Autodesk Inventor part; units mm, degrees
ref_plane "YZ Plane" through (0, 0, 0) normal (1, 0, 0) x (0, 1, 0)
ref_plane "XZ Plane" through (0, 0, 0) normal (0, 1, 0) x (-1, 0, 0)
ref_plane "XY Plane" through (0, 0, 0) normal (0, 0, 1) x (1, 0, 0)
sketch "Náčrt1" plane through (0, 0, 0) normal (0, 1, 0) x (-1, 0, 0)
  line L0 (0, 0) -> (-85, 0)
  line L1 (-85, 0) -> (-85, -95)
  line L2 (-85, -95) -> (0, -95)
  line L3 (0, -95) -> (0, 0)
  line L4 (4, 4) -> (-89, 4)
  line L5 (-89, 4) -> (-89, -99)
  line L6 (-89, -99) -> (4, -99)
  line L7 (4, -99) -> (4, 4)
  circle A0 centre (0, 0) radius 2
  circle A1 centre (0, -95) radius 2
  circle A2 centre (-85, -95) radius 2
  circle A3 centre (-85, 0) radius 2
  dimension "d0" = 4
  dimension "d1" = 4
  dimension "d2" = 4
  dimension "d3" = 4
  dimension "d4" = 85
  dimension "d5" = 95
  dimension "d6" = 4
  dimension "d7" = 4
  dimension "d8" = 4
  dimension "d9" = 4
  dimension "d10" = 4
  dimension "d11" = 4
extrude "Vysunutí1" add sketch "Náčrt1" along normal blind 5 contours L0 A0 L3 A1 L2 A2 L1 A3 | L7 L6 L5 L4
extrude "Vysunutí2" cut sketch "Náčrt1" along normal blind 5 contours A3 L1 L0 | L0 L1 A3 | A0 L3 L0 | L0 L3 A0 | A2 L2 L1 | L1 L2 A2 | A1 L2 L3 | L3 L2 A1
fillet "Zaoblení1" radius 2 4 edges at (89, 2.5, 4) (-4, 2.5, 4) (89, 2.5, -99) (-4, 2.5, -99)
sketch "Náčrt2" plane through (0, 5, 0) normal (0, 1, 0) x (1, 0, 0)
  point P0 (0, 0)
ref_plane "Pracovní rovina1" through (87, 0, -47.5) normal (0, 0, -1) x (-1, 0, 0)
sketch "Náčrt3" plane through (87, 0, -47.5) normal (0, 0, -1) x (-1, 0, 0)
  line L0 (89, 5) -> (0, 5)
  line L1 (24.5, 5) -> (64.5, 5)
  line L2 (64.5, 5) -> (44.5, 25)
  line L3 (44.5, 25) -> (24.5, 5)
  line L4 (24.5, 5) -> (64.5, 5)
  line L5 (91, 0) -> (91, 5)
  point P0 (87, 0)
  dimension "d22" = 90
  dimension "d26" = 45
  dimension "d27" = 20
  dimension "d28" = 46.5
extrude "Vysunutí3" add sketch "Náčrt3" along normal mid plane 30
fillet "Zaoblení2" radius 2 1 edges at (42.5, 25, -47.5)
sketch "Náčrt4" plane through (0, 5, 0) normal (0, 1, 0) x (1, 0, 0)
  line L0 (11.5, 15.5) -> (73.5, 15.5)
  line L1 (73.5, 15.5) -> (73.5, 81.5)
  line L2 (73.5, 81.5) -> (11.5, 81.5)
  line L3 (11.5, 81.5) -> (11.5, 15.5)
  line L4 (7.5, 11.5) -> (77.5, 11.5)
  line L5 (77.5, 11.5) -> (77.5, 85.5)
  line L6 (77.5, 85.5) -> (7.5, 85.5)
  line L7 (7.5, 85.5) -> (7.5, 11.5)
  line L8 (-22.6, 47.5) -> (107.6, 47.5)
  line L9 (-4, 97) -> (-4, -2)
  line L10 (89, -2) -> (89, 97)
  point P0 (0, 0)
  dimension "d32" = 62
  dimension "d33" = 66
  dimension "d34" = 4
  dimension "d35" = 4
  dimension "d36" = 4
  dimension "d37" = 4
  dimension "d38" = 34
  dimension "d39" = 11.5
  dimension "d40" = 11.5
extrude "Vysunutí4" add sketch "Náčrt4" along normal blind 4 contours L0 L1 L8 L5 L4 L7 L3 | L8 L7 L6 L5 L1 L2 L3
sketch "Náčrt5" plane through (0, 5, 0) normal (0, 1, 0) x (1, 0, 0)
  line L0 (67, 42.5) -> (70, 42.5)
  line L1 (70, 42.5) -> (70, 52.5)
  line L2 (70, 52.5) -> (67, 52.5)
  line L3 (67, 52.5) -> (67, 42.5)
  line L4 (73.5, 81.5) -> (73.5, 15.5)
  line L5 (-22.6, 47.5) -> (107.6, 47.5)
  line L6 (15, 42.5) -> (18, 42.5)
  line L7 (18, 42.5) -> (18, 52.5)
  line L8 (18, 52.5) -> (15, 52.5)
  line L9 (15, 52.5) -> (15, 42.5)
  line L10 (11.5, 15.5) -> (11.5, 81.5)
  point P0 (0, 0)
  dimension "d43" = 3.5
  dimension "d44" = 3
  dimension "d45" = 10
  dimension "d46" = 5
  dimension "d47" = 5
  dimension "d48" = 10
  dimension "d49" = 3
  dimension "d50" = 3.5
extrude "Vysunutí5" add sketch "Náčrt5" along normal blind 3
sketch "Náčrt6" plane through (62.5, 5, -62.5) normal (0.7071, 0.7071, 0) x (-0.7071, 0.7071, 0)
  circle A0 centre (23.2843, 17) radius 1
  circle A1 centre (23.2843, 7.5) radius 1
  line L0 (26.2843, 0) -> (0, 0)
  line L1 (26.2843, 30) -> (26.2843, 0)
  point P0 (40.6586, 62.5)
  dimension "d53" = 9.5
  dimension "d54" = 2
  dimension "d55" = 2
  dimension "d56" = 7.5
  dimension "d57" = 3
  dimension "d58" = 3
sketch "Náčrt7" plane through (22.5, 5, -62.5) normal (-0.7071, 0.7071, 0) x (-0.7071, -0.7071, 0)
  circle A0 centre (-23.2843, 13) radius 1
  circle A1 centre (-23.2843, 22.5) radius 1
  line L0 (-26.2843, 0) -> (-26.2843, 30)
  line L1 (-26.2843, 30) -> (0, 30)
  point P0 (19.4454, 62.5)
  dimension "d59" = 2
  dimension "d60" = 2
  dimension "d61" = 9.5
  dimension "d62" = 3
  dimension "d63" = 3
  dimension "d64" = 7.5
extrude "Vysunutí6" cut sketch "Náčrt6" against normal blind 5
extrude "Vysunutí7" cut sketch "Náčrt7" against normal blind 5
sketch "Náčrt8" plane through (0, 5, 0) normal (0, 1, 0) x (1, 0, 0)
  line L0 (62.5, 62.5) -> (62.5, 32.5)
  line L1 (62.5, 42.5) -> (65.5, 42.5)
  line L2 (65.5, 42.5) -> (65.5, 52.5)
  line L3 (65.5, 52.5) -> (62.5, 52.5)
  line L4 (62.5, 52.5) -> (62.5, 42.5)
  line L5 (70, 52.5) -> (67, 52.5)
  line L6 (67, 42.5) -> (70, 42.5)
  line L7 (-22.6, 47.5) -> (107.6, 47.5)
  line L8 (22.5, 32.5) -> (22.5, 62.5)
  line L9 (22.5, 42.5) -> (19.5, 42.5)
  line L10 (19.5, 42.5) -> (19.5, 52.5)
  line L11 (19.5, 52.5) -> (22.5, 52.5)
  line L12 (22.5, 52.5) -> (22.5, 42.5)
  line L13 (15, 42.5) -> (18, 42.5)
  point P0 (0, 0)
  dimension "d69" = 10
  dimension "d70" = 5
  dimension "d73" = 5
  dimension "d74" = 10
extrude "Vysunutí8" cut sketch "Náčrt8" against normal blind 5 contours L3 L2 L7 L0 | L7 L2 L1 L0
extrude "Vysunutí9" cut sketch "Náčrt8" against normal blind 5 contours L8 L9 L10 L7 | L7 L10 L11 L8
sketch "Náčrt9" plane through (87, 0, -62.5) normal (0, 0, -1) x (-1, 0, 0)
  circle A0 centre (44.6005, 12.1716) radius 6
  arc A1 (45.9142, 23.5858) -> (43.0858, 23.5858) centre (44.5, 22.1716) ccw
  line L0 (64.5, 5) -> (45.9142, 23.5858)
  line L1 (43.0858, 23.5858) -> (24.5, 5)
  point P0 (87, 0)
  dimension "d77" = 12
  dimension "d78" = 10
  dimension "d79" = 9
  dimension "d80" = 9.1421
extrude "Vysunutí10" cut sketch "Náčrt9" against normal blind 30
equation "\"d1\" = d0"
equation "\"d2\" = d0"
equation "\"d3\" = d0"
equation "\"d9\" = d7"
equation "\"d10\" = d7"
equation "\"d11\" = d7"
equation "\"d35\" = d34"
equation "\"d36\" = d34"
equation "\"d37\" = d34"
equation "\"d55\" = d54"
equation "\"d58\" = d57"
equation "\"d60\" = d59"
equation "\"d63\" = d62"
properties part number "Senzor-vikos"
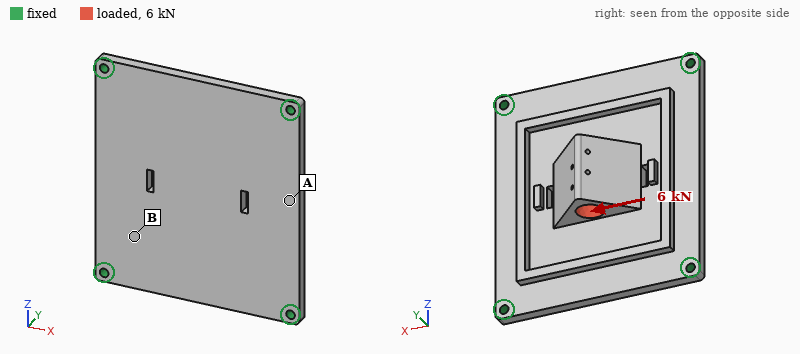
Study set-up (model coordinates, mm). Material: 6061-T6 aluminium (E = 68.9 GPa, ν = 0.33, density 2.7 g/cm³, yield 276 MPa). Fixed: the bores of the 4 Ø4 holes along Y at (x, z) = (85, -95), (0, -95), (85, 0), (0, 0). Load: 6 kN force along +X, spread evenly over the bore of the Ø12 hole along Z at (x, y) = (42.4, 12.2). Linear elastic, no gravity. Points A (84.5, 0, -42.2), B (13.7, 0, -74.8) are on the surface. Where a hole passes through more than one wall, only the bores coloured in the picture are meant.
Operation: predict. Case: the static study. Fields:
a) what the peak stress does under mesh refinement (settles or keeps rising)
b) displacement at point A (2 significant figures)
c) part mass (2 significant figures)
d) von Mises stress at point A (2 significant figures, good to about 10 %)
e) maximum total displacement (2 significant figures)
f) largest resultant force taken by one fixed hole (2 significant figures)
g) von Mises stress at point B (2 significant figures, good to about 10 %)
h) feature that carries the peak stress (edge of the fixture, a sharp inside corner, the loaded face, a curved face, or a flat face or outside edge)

keeps rising
91 µm
160 g
32 MPa
97 µm
1.9 kN
14 MPa
edge of the fixture
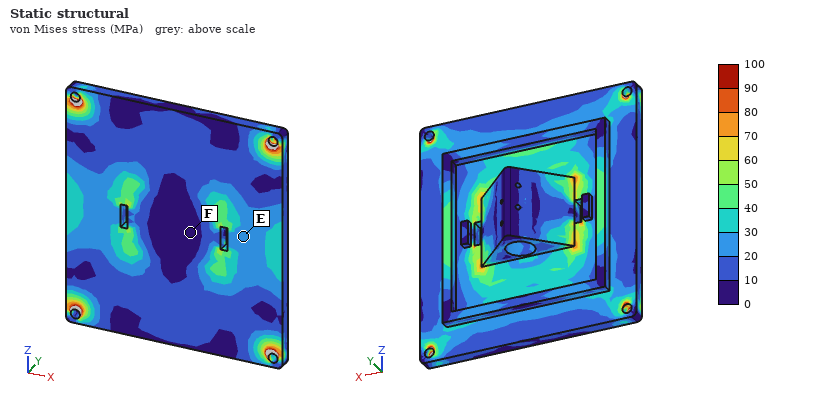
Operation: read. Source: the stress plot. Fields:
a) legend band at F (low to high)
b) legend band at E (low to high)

0 to 10 MPa
20 to 30 MPa
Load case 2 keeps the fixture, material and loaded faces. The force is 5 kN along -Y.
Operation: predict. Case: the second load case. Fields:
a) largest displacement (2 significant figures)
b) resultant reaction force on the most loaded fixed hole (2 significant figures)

0.41 mm
1.6 kN
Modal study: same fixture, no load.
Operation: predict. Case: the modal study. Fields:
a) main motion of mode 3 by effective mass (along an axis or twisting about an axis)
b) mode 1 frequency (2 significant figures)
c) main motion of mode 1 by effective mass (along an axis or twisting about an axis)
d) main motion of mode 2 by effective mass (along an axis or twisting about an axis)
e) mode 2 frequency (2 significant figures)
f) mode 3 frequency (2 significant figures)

twisting about X
1900 Hz
along Y
twisting about Z
3300 Hz
3700 Hz
